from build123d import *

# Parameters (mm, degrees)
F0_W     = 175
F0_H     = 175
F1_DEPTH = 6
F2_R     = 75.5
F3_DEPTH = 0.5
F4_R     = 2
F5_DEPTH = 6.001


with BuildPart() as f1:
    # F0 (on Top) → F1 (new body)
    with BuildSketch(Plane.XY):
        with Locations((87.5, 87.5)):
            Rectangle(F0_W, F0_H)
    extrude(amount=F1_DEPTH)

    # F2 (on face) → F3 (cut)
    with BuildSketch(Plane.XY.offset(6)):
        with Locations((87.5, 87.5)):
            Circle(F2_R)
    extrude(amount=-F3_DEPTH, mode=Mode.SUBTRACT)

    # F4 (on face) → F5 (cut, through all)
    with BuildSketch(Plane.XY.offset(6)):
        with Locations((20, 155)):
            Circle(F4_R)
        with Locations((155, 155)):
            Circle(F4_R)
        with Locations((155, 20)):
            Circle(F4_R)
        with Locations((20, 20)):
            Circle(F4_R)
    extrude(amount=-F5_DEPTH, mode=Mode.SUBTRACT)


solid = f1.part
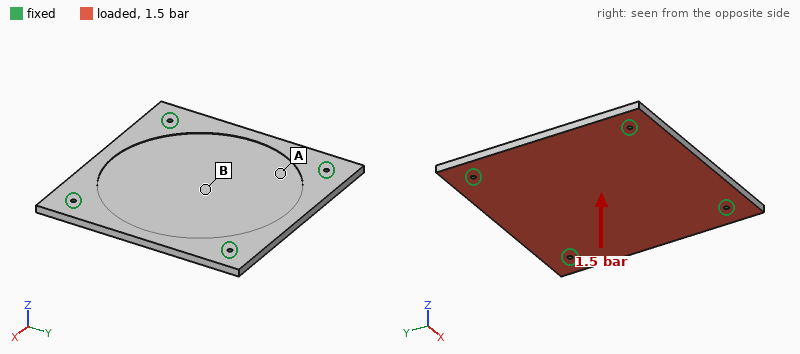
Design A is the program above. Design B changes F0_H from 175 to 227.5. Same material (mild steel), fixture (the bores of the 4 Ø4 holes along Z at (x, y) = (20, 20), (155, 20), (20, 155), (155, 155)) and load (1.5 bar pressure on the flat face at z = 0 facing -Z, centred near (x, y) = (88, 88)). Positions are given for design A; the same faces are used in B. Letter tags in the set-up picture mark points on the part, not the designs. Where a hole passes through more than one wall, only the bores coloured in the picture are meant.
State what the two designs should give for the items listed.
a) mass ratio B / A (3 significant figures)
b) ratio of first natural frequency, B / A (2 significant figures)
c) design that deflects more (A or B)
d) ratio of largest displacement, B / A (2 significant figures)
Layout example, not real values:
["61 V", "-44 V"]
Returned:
["1.32", "1.0", "A", "0.90"]
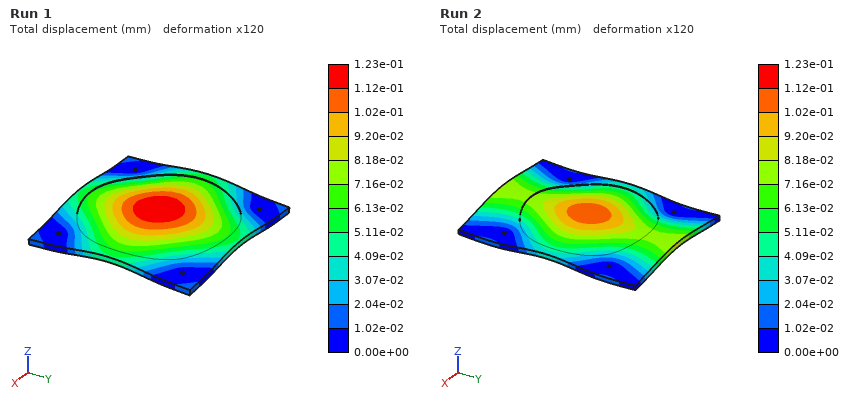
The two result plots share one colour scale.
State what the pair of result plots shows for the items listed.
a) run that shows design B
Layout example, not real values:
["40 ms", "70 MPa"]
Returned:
["Run 2"]
